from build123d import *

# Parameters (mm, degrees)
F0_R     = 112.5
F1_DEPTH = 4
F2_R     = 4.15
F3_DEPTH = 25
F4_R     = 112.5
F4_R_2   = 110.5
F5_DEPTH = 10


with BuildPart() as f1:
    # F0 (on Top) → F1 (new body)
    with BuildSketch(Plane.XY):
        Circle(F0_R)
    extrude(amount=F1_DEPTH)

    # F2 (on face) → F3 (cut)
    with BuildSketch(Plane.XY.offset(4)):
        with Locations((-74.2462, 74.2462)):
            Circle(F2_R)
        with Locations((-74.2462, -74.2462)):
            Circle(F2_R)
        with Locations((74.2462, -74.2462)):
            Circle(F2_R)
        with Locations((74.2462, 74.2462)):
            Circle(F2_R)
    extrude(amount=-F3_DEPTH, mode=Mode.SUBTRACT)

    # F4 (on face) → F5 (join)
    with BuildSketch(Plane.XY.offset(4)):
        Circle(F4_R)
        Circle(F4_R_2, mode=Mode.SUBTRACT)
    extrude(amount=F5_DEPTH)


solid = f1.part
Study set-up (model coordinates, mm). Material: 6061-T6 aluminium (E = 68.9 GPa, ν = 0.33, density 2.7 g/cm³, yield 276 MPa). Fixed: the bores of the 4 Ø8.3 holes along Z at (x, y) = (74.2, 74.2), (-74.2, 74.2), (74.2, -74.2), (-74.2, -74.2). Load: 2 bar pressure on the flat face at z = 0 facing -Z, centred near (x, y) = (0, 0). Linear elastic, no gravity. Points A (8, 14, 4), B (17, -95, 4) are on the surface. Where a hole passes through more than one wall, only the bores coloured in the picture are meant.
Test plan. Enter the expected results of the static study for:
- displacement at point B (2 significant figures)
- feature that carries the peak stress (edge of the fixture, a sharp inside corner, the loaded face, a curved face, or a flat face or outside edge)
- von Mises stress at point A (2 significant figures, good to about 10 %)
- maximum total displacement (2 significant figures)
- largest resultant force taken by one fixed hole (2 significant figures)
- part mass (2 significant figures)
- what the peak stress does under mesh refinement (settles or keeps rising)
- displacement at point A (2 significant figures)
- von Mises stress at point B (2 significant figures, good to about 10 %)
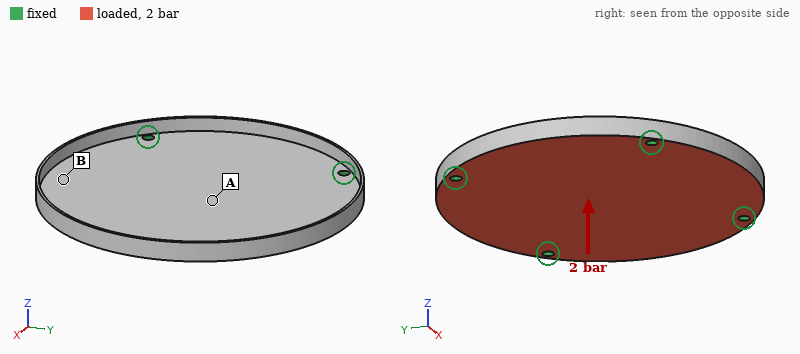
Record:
0.33 mm
edge of the fixture
79 MPa
1.5 mm
2.0 kN
460 g
keeps rising
1.4 mm
39 MPa
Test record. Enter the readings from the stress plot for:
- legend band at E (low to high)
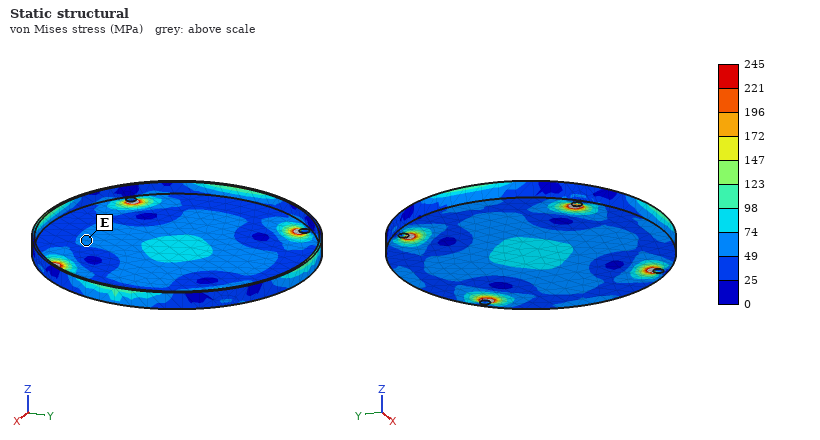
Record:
49 to 74 MPa
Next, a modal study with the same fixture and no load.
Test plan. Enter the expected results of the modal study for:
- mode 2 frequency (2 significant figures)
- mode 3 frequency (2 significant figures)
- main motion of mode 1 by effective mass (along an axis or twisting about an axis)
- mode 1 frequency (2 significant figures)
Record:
1200 Hz
1300 Hz
along Z
710 Hz
